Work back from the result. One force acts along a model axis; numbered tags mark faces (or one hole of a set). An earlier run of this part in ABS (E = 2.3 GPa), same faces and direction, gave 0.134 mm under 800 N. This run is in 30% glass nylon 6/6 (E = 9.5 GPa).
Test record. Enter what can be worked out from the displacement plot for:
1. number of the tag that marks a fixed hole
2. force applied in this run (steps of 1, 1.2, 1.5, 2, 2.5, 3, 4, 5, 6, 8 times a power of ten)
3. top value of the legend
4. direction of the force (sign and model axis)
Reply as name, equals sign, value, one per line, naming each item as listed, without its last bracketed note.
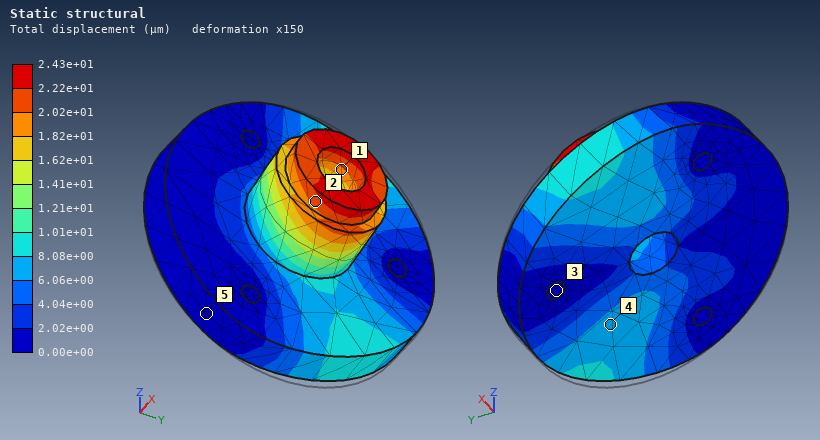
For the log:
number of the tag that marks a fixed hole = 3
force applied in this run = 600 N
top value of the legend = 2.43e+01 µm
direction of the force = +Z
